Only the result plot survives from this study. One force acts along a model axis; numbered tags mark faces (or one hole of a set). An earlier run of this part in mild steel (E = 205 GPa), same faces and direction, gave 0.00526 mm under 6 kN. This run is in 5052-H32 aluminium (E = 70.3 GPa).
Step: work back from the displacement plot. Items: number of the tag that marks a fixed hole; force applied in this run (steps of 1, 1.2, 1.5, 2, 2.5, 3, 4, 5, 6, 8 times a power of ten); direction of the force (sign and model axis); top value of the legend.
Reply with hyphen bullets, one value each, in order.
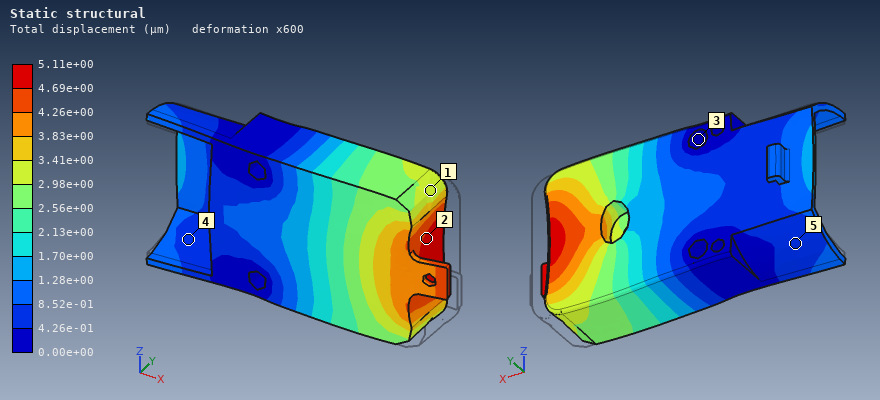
- 3
- 2 kN
- -X
- 5.11e+00 µm
